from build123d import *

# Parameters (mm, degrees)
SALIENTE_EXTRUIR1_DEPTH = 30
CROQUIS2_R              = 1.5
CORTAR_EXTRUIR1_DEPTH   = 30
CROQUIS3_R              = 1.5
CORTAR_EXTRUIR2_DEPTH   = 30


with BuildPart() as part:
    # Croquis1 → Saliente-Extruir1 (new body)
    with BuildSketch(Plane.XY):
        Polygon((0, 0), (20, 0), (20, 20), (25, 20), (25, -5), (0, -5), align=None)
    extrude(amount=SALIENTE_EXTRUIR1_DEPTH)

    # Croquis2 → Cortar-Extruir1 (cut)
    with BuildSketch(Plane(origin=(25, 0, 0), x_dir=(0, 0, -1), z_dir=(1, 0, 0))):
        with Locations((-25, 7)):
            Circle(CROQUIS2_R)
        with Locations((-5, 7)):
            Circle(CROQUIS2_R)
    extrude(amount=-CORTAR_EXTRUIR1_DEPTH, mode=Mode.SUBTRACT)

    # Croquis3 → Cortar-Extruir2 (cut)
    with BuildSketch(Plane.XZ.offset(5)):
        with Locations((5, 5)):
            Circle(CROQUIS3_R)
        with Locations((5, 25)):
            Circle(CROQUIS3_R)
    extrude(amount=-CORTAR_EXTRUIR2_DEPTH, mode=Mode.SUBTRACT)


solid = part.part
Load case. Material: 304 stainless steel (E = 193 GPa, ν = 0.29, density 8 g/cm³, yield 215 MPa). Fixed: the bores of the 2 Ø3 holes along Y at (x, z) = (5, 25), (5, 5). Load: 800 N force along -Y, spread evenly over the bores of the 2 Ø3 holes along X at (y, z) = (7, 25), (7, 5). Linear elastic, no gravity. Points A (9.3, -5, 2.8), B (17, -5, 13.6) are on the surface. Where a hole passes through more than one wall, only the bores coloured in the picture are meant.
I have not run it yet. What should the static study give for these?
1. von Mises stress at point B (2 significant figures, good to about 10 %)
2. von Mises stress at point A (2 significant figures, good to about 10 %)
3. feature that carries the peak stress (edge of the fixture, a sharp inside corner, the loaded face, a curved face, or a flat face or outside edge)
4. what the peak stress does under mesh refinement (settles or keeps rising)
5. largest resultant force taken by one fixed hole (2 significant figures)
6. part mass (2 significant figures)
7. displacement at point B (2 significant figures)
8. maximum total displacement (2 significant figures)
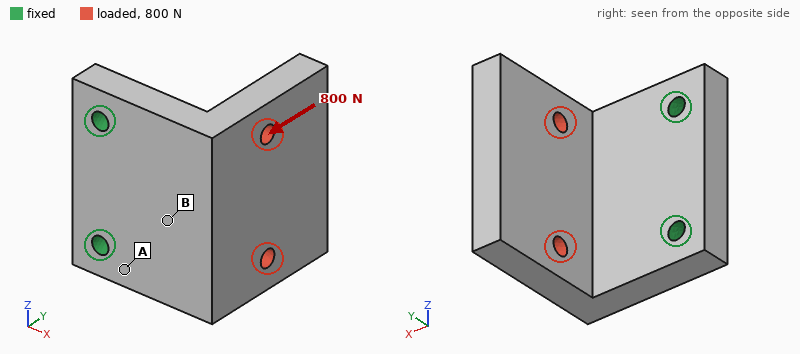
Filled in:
32 MPa
95 MPa
edge of the fixture
keeps rising
400 N
53 g
18 µm
61 µm
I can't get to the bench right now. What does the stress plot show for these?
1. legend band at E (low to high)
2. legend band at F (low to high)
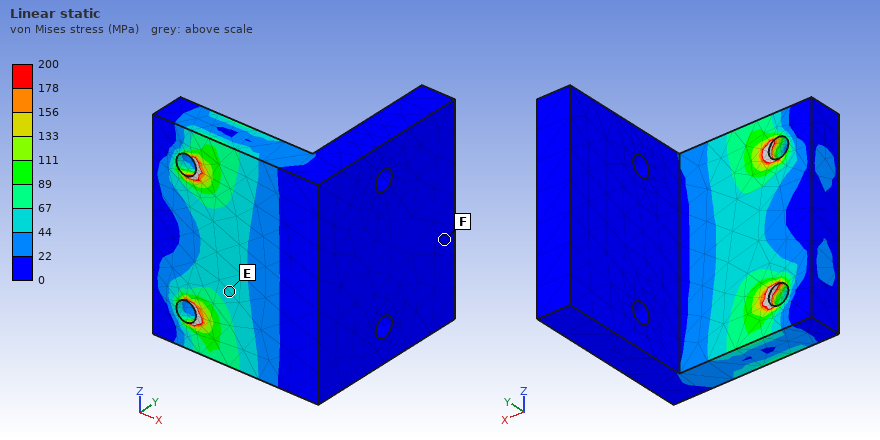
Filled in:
44 to 67 MPa
0 to 22 MPa
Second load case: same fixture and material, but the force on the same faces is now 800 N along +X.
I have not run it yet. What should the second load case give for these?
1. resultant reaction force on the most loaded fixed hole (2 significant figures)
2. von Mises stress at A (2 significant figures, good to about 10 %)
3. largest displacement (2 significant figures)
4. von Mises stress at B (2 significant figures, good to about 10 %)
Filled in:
410 N
60 MPa
64 µm
49 MPa
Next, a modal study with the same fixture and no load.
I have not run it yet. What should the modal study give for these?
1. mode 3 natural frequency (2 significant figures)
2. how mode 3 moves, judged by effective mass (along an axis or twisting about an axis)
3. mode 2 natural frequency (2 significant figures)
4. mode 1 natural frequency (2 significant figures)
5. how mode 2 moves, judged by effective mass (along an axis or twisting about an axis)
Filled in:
8800 Hz
along Y
5800 Hz
3200 Hz
along Z
